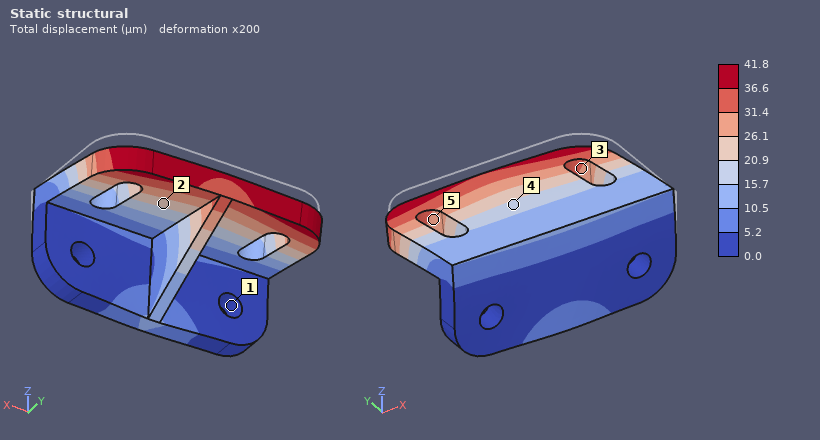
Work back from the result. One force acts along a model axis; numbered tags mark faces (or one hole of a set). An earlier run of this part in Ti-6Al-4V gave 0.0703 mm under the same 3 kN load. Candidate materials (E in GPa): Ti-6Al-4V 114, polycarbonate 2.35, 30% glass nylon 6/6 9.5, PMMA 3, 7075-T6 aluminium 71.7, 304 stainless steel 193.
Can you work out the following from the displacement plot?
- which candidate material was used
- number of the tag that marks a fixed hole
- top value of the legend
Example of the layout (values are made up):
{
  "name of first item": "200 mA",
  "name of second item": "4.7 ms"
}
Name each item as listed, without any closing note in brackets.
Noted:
{
  "which candidate material was used": "304 stainless steel",
  "number of the tag that marks a fixed hole": "1",
  "top value of the legend": "41.8 µm"
}
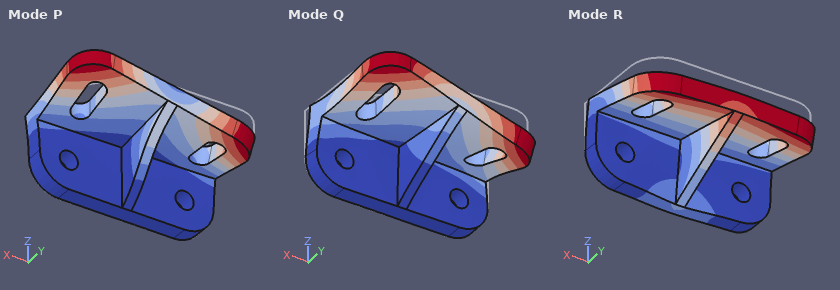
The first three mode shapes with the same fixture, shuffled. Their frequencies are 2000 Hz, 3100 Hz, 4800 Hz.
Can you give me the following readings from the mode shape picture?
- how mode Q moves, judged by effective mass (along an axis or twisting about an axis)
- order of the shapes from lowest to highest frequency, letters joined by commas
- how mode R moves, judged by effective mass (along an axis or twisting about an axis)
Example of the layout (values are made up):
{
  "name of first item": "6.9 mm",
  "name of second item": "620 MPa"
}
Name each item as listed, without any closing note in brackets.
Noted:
{
  "how mode Q moves, judged by effective mass": "along X",
  "order of the shapes from lowest to highest frequency, letters joined by commas": "R, P, Q",
  "how mode R moves, judged by effective mass": "along Z"
}
